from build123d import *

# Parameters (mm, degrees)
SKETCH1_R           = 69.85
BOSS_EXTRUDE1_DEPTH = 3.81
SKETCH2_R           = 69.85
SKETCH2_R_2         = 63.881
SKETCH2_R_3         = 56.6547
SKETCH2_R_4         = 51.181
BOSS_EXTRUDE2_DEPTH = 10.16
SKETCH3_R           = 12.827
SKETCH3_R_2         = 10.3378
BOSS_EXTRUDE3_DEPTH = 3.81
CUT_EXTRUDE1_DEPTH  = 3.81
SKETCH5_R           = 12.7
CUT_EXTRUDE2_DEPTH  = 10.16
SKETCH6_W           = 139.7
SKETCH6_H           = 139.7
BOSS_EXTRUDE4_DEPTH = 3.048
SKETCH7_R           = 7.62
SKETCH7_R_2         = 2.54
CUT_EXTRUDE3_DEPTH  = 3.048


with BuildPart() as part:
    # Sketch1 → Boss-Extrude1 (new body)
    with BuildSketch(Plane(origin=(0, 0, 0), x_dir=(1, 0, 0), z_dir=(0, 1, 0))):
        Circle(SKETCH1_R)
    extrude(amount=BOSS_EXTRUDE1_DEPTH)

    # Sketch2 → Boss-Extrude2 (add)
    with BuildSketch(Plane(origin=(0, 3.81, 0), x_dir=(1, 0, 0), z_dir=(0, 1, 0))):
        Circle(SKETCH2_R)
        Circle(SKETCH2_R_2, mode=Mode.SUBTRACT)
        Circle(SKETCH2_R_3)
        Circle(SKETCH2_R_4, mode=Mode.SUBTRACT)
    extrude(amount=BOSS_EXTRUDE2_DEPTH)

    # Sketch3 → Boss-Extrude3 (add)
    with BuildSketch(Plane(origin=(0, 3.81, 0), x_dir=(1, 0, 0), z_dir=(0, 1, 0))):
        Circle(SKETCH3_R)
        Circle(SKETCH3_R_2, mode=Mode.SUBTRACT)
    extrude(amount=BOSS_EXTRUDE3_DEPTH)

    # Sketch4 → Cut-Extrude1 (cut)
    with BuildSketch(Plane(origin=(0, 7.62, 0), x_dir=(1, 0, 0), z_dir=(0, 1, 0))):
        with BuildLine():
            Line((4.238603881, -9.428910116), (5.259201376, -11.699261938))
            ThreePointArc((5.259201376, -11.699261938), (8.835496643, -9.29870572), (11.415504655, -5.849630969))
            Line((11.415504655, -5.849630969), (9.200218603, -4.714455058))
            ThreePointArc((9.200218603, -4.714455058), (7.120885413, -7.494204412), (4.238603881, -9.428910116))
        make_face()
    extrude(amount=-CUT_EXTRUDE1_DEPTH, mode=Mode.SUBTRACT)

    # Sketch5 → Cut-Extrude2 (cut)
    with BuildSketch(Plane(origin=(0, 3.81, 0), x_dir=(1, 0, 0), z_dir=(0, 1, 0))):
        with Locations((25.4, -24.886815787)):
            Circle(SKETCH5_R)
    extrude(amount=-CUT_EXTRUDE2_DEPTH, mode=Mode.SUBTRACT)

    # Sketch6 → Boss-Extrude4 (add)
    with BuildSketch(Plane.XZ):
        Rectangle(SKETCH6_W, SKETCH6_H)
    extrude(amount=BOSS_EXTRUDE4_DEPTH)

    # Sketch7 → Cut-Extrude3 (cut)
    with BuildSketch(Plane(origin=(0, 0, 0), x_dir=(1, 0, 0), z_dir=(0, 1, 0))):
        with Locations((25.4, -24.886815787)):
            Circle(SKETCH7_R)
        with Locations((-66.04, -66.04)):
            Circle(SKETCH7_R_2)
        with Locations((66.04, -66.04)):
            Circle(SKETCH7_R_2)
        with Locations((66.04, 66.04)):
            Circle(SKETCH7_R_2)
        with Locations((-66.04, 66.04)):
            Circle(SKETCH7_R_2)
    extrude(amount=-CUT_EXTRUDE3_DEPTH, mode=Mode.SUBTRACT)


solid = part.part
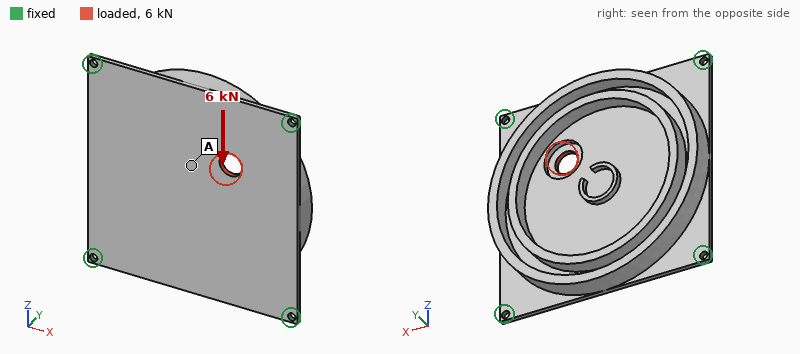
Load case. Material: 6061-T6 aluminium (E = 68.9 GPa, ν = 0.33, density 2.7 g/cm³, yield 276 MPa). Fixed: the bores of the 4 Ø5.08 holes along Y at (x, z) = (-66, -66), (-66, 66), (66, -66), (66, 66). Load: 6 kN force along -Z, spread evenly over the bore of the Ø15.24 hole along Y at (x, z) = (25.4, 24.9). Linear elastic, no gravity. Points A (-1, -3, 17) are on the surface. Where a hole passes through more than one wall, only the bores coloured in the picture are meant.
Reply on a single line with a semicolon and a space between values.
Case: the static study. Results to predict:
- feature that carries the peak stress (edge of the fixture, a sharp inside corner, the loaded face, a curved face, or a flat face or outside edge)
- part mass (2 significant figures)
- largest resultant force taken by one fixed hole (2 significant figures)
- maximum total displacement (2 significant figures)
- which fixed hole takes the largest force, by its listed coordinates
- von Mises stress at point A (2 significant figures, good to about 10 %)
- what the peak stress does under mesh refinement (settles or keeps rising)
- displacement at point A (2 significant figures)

edge of the fixture; 430 g; 2.1 kN; 32 µm; (66, 66); 7.5 MPa; keeps rising; 19 µm
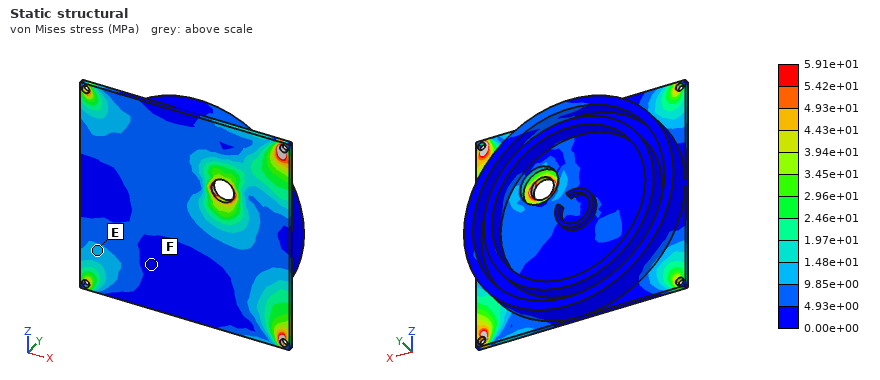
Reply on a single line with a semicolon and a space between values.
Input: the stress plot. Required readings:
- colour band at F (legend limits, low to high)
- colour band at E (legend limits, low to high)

0.00e+00 to 4.93e+00 MPa; 9.85e+00 to 1.48e+01 MPa
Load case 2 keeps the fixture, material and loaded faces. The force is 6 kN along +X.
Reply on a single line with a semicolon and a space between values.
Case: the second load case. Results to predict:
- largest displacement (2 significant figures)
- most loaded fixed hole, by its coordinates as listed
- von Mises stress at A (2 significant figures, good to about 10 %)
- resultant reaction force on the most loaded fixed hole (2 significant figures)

32 µm; (66, 66); 13 MPa; 2.1 kN
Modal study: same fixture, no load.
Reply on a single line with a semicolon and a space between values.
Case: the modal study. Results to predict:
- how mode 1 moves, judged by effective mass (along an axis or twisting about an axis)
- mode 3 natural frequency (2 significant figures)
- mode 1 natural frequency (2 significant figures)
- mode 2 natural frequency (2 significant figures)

along Y; 1300 Hz; 830 Hz; 1200 Hz
